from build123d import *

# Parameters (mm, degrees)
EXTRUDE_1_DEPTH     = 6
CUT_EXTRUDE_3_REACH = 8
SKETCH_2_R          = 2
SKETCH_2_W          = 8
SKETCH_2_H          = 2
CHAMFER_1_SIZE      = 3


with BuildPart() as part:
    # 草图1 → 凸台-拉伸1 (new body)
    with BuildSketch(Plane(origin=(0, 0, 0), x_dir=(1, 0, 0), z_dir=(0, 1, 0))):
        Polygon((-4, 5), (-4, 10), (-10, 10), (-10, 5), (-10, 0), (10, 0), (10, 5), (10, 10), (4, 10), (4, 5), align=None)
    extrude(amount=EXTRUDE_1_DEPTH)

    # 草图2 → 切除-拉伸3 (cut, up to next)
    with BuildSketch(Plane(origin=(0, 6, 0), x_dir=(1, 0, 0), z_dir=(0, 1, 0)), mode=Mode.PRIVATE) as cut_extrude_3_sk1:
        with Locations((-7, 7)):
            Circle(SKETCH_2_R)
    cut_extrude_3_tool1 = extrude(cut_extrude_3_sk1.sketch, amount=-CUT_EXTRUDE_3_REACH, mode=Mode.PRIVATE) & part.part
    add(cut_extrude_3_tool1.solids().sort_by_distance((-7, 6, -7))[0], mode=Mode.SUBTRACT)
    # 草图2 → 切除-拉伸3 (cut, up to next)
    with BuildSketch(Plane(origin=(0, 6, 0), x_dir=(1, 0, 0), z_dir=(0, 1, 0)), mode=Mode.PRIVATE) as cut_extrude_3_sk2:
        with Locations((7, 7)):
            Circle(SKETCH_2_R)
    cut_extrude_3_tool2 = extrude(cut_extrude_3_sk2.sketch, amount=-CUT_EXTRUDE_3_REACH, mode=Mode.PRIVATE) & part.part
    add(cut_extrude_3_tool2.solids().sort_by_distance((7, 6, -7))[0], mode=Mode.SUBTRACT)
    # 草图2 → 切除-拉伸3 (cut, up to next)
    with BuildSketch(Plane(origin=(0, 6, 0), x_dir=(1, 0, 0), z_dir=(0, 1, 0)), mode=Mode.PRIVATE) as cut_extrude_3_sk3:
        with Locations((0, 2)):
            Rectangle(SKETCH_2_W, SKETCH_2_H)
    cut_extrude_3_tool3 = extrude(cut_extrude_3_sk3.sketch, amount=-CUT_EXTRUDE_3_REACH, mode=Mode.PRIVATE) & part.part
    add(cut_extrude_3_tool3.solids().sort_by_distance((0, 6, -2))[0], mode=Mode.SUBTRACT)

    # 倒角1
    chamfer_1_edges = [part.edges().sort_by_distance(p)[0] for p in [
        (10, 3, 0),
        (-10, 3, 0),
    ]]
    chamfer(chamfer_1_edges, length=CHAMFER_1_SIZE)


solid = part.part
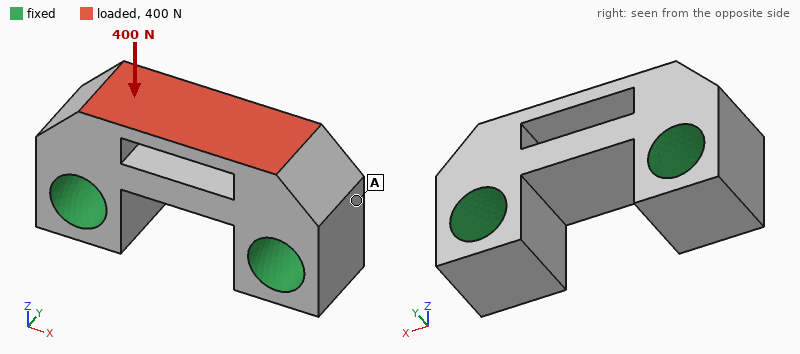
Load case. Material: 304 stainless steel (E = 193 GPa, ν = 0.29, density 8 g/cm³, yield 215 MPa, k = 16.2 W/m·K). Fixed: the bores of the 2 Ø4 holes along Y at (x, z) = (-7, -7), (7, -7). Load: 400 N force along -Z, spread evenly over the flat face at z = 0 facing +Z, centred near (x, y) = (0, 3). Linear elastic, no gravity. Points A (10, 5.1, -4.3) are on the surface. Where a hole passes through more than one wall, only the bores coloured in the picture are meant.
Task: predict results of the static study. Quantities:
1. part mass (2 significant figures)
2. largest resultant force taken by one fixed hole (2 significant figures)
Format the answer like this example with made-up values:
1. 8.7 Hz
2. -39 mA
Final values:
1. 5.3 g
2. 220 N
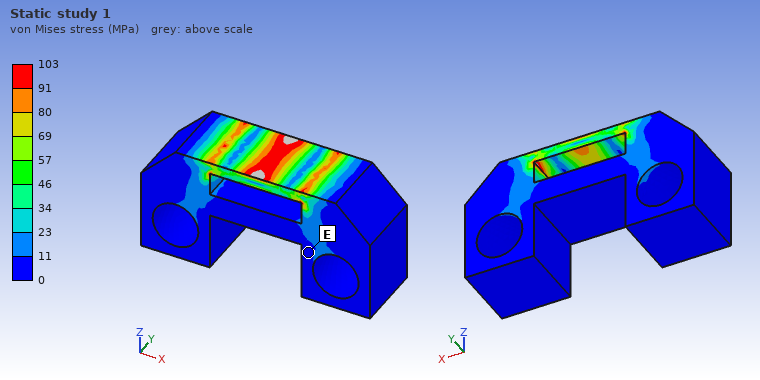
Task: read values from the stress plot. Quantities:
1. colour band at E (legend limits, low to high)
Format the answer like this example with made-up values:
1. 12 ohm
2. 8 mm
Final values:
1. 0 to 11 MPa
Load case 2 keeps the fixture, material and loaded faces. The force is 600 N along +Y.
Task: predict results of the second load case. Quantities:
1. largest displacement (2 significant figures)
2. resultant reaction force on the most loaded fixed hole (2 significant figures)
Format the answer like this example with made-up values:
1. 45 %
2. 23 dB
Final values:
1. 5.5 µm
2. 300 N
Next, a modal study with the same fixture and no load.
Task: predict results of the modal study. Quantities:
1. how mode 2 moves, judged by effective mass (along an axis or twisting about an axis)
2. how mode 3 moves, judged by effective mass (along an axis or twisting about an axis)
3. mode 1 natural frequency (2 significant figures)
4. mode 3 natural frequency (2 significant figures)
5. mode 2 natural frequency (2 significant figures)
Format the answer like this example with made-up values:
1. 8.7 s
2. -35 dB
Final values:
1. along Y
2. along Y
3. 57 kHz
4. 79 kHz
5. 73 kHz
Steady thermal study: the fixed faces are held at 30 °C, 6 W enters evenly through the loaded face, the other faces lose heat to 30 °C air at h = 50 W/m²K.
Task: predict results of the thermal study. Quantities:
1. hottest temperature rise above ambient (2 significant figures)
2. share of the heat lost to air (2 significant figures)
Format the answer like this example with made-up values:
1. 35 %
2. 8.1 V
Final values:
1. 79 K
2. 7.0 %
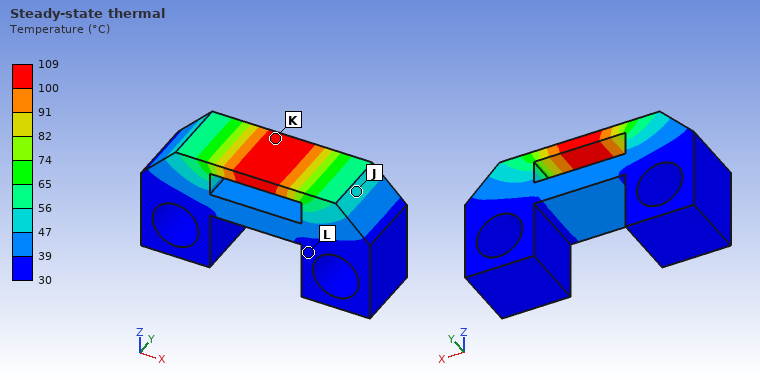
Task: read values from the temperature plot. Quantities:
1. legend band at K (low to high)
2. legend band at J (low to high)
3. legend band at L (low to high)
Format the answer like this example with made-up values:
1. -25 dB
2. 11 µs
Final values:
1. 100 to 109 °C
2. 47 to 56 °C
3. 30 to 39 °C
